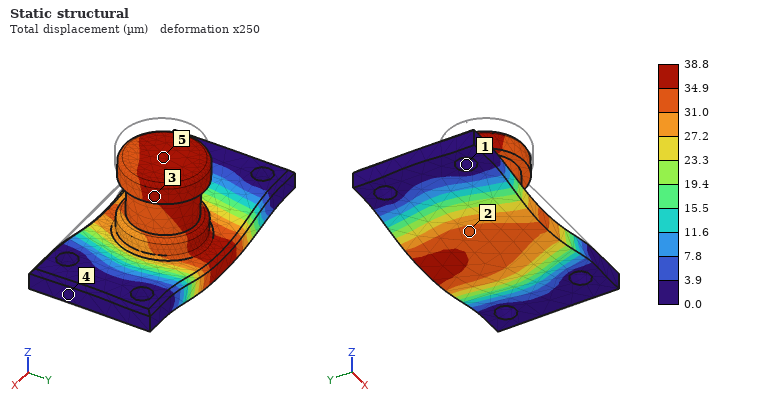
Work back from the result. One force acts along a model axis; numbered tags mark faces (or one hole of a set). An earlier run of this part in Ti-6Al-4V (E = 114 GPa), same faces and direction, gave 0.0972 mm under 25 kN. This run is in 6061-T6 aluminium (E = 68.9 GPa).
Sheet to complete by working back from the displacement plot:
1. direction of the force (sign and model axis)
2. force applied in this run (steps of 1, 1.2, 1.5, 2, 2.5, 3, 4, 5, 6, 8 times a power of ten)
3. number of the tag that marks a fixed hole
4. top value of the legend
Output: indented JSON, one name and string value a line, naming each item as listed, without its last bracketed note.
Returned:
{
  "direction of the force": "-Z",
  "force applied in this run": "6 kN",
  "number of the tag that marks a fixed hole": "1",
  "top value of the legend": "38.8 µm"
}
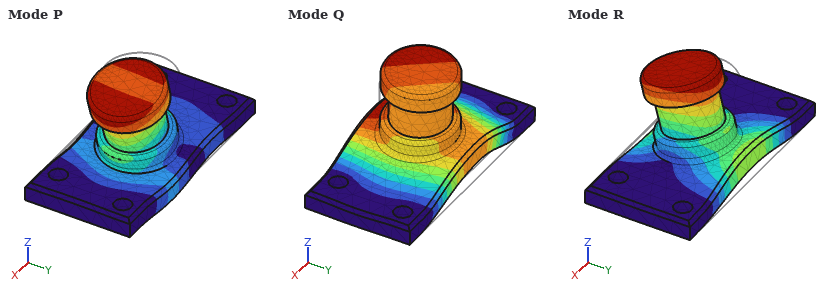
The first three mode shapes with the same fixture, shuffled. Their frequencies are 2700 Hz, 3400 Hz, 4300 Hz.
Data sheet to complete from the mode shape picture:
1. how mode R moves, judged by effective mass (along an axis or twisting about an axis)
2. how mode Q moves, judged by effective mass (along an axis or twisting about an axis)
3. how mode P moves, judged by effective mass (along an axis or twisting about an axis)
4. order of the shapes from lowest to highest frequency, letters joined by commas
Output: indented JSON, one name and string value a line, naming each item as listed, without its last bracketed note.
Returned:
{
  "how mode R moves, judged by effective mass": "along Y",
  "how mode Q moves, judged by effective mass": "along Z",
  "how mode P moves, judged by effective mass": "along X",
  "order of the shapes from lowest to highest frequency, letters joined by commas": "R, Q, P"
}
